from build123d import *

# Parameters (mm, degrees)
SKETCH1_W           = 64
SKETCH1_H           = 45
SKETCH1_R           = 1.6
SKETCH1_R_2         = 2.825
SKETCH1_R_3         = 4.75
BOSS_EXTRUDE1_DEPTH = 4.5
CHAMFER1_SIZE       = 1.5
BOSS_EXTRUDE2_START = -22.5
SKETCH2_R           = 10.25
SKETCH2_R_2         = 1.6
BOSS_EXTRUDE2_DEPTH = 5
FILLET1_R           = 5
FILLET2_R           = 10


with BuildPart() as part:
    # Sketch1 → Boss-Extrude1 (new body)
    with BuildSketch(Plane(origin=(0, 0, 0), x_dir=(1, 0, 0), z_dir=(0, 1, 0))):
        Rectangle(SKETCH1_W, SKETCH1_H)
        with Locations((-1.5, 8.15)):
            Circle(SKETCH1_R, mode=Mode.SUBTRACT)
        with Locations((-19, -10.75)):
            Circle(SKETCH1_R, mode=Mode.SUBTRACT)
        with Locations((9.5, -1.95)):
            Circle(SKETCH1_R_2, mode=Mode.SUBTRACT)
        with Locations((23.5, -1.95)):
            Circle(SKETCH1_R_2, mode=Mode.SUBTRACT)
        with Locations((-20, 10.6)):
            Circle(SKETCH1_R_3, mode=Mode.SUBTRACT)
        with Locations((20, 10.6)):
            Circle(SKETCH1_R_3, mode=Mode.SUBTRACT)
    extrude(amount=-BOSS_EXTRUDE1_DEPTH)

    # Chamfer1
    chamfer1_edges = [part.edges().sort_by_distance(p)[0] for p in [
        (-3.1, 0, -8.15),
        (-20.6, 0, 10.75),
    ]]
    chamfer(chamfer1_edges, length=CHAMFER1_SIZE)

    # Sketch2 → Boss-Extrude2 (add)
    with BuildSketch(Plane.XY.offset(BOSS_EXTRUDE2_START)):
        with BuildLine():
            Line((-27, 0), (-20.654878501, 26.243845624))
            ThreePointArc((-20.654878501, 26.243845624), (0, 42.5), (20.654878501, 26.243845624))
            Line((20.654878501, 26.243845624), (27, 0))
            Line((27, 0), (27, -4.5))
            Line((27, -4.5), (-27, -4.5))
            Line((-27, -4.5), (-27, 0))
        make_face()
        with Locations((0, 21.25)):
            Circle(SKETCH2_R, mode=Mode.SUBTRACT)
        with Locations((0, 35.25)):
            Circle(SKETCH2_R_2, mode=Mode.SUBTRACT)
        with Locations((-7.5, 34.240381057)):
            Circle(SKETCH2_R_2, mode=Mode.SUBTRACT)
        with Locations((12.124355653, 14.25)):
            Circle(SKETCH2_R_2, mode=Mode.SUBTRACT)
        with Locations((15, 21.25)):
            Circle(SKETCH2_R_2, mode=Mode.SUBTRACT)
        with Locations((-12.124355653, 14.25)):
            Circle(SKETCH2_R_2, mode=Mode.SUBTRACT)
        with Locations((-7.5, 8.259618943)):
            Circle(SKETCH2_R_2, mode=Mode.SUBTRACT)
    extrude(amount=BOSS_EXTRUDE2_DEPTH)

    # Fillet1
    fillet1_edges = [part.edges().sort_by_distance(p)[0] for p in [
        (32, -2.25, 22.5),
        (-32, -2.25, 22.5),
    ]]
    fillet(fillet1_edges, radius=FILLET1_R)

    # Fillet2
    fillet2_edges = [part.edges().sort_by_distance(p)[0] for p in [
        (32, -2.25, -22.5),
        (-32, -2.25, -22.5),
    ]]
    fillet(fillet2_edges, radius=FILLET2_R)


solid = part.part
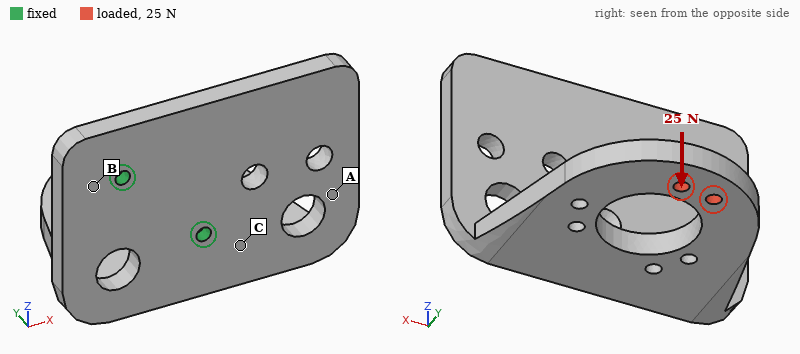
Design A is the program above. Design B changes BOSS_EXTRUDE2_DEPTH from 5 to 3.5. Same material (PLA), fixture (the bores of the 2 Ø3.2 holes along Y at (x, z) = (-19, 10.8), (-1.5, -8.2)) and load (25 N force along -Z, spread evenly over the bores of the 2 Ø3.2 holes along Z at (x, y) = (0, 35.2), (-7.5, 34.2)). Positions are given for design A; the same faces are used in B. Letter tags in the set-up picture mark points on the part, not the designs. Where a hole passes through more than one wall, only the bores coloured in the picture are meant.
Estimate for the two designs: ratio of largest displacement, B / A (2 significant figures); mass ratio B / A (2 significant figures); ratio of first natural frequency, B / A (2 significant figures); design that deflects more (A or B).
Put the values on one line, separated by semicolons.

1.8; 0.89; 0.98; B
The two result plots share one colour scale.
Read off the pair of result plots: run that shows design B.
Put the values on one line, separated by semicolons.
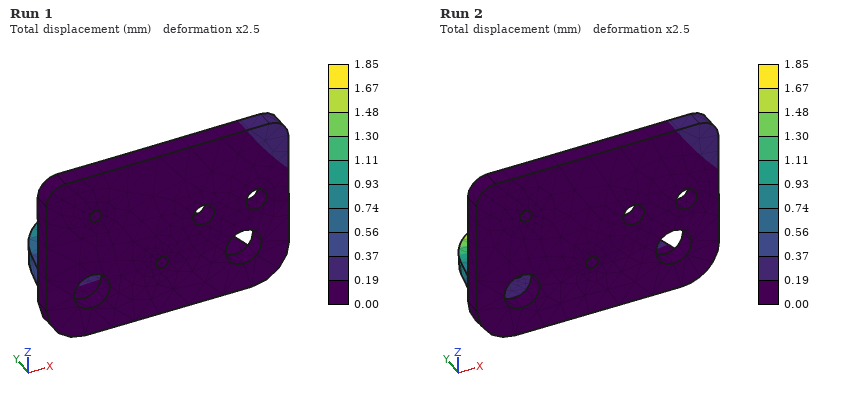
Run 2
